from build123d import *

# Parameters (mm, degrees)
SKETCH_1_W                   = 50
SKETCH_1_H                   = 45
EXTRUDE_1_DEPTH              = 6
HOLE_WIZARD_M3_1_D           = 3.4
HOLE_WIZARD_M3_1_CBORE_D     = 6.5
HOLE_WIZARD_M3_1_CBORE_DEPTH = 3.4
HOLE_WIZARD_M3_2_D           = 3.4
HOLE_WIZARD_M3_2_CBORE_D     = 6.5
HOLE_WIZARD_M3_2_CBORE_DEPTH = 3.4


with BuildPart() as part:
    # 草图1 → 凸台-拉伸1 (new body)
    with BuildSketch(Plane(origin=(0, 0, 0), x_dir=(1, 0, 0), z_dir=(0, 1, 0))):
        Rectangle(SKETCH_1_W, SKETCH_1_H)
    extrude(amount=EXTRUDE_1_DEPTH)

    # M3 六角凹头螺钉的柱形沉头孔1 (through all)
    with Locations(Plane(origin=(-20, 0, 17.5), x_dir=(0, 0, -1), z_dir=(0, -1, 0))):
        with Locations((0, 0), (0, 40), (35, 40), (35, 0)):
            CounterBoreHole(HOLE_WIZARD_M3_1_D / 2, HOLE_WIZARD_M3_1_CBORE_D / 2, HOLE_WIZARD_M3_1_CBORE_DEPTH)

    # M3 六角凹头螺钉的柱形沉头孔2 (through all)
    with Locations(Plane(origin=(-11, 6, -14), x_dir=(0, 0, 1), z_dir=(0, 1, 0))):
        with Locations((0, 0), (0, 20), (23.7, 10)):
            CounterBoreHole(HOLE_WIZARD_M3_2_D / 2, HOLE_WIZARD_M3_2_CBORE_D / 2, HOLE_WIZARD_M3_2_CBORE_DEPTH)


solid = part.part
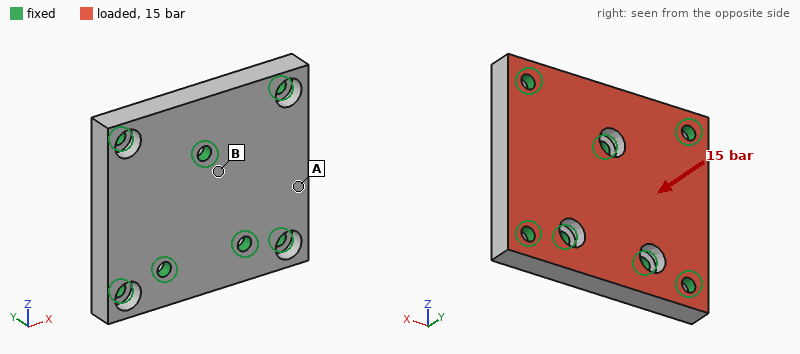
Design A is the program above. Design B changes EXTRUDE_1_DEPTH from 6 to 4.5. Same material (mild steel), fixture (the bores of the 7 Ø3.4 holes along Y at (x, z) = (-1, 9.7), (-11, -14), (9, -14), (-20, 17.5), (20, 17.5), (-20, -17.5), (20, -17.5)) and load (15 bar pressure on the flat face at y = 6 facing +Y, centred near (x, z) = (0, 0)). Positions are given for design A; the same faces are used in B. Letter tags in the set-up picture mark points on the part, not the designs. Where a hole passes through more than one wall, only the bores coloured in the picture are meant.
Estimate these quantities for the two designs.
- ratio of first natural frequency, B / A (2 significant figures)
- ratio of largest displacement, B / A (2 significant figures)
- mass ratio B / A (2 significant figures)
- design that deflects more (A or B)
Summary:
0.77
2.4
0.75
B
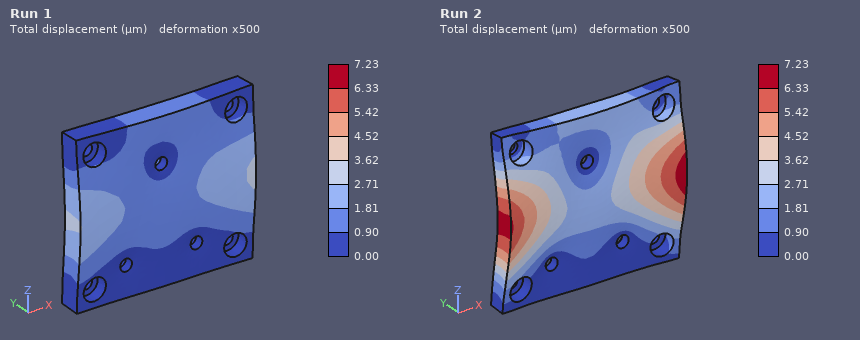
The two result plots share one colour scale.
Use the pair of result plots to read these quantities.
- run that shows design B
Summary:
Run 2
